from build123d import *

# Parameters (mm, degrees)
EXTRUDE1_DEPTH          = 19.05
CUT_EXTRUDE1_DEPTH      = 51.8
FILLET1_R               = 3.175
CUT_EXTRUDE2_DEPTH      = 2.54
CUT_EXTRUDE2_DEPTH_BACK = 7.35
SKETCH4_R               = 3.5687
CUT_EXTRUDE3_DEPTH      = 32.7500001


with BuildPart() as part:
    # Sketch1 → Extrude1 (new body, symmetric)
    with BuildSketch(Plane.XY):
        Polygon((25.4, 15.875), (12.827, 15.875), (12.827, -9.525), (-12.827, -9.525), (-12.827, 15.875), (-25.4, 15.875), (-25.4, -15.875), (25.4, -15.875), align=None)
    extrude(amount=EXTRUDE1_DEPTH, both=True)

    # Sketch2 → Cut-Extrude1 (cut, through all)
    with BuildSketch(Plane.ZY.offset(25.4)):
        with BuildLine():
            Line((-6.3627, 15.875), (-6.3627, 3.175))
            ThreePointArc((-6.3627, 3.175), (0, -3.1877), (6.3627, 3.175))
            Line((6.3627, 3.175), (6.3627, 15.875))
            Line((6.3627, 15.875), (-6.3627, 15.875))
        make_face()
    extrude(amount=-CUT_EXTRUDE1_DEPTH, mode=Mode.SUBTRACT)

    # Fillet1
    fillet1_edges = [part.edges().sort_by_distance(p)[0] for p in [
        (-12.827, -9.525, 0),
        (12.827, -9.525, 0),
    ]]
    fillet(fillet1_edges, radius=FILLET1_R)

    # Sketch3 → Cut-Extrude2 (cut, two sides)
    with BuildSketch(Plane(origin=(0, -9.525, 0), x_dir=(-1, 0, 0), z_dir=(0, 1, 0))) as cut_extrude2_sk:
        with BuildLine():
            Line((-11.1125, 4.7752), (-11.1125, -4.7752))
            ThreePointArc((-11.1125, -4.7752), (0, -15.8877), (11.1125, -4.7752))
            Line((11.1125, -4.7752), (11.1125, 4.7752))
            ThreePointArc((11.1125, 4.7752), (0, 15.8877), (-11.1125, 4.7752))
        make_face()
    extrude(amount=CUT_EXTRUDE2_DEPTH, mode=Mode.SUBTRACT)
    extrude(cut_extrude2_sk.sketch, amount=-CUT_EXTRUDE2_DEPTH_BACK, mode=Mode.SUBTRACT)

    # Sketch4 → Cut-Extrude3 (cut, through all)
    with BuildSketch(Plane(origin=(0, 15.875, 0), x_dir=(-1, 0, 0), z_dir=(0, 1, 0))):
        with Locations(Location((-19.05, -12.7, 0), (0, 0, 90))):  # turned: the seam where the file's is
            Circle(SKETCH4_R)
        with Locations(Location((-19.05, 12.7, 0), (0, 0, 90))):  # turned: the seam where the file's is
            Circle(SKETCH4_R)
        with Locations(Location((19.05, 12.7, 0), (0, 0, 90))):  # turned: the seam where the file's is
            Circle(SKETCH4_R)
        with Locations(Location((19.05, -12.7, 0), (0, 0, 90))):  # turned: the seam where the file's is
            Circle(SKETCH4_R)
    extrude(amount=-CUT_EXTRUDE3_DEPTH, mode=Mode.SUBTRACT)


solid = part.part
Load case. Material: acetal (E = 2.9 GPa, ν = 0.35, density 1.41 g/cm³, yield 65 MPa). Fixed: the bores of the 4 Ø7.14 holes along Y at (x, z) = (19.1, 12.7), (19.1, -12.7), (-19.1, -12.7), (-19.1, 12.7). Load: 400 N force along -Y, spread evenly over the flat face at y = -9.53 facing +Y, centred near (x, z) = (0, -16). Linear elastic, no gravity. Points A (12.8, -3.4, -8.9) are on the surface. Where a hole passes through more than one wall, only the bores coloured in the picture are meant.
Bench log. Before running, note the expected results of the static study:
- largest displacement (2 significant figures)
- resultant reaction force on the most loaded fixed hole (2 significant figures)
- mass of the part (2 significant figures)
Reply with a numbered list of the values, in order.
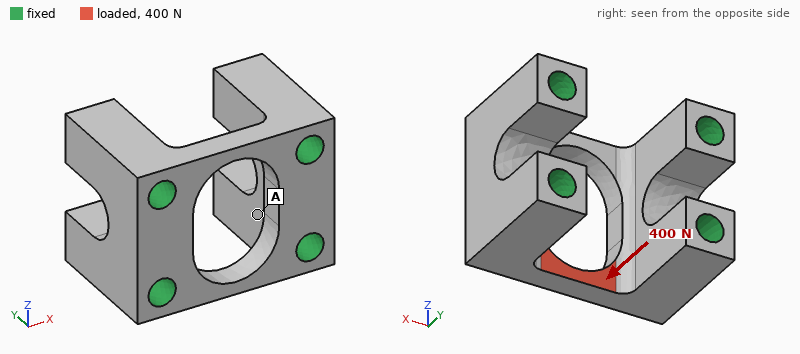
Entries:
1. 0.13 mm
2. 210 N
3. 31 g
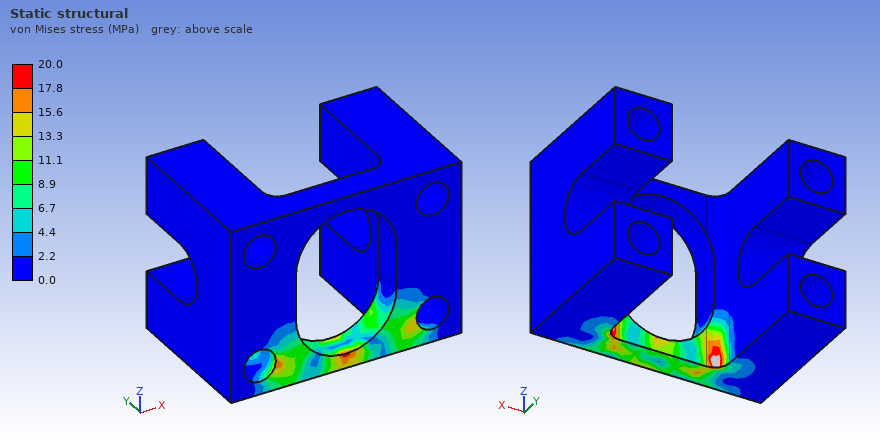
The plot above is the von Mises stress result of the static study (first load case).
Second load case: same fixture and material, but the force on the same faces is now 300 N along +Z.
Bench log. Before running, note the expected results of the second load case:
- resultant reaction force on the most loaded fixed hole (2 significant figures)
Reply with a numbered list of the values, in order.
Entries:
1. 130 N
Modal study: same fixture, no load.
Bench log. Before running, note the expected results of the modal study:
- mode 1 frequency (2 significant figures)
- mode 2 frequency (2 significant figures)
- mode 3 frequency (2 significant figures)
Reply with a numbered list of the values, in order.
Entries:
1. 11 kHz
2. 11 kHz
3. 13 kHz
